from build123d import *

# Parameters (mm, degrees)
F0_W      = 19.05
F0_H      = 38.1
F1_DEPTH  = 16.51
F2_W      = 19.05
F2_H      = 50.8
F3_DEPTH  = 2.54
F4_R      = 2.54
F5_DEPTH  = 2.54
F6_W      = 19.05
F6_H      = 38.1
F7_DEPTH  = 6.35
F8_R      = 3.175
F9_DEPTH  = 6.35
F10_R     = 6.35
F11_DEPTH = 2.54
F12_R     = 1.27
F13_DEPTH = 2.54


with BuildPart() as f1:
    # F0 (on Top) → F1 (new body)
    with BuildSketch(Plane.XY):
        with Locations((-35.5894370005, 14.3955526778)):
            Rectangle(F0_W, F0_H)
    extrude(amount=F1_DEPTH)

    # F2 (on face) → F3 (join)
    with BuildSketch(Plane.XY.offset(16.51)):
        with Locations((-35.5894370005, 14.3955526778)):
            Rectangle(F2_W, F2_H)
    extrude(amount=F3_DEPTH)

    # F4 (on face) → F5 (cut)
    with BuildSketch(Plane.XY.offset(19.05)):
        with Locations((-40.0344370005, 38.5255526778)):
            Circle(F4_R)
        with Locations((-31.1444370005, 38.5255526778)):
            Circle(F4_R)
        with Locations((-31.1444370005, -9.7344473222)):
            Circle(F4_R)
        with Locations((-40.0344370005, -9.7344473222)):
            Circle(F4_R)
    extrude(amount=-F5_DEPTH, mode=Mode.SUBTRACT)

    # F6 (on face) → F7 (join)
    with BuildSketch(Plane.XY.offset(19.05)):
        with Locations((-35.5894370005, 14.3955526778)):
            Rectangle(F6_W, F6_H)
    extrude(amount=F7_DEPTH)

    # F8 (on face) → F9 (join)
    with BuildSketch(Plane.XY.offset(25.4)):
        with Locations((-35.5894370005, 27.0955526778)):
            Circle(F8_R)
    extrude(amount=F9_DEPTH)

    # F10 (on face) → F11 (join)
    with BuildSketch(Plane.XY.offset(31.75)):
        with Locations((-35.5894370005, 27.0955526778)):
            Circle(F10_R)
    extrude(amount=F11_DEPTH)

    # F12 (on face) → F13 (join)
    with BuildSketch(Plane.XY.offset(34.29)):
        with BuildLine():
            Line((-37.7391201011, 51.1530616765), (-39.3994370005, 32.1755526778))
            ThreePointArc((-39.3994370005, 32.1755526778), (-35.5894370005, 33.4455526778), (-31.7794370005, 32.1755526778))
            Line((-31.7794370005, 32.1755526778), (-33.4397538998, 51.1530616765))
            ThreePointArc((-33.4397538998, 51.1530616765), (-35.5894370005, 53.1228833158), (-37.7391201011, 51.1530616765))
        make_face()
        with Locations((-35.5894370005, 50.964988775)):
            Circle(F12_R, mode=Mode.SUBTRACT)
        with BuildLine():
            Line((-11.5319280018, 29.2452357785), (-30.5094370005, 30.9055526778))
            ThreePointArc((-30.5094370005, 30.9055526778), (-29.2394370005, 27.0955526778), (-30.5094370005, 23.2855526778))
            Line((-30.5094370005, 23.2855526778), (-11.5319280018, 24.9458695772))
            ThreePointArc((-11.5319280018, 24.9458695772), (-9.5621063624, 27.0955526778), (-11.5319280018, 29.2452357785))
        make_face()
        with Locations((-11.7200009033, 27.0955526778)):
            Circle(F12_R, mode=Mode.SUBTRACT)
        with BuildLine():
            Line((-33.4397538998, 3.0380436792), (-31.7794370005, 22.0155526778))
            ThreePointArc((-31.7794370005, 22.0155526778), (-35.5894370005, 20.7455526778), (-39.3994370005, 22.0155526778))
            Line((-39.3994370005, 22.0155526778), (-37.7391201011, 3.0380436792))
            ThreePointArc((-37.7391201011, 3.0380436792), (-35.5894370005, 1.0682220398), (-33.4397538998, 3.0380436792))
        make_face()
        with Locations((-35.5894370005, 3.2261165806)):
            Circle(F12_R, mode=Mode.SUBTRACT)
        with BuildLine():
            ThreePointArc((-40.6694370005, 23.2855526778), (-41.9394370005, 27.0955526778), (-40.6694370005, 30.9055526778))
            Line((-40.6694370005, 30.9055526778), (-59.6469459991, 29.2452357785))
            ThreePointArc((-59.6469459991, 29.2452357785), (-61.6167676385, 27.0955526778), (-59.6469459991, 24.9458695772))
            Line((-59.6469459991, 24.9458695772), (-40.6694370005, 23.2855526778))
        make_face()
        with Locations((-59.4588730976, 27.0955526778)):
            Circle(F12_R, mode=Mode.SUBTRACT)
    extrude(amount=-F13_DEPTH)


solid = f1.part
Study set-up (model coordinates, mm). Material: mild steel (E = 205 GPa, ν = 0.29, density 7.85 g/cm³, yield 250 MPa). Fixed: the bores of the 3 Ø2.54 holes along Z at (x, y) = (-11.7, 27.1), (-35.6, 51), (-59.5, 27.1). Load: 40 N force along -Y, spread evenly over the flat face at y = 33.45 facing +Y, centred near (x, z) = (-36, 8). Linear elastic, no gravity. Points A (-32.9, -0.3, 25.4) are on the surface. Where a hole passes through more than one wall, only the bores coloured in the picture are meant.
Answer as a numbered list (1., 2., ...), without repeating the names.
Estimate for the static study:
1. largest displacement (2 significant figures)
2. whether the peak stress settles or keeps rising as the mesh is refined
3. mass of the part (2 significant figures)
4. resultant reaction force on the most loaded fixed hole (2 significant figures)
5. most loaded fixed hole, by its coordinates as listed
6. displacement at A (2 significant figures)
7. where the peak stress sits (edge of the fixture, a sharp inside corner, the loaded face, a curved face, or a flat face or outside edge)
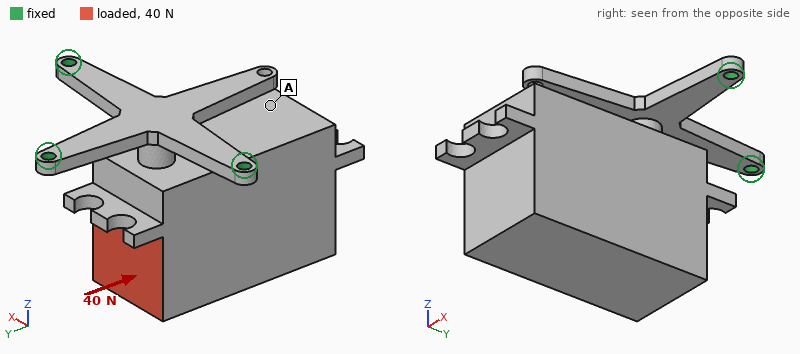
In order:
1. 0.11 mm
2. keeps rising
3. 160 g
4. 51 N
5. (-35.6, 51)
6. 0.074 mm
7. edge of the fixture
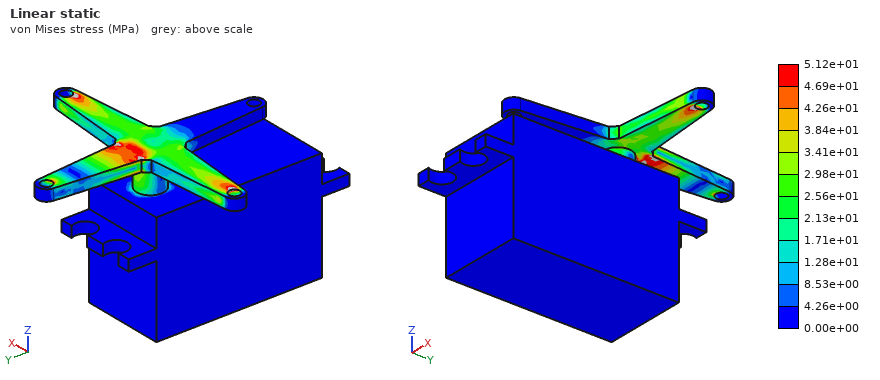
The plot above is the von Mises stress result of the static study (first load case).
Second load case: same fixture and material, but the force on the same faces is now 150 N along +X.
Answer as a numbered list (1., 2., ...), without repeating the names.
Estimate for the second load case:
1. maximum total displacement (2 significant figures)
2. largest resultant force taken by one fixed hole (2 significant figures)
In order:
1. 0.17 mm
2. 120 N
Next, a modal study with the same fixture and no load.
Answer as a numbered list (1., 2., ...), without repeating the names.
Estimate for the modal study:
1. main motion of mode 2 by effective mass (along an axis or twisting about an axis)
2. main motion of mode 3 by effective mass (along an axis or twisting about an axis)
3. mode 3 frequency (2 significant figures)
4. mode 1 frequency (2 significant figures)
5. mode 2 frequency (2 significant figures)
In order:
1. along X
2. twisting about Z
3. 1200 Hz
4. 290 Hz
5. 480 Hz
